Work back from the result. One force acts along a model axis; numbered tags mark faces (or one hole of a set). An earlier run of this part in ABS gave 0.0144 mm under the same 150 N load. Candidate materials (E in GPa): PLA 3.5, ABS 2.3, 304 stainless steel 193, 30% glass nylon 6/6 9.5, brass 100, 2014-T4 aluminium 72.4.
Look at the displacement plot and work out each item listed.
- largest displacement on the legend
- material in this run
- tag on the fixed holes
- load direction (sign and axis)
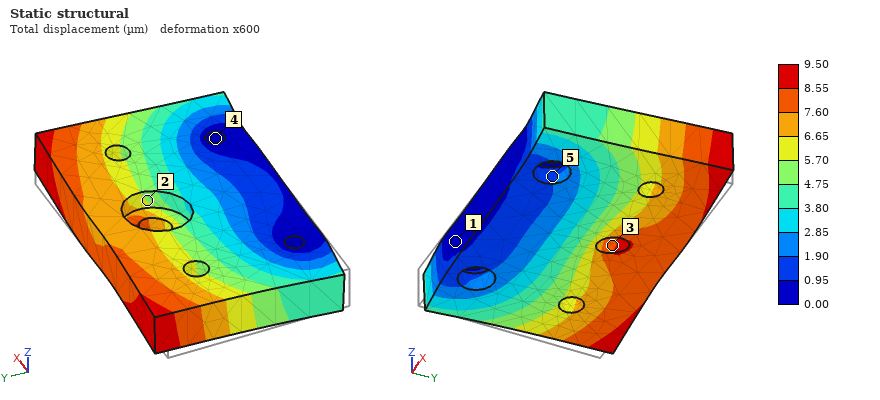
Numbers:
9.50 µm
PLA
4
+X
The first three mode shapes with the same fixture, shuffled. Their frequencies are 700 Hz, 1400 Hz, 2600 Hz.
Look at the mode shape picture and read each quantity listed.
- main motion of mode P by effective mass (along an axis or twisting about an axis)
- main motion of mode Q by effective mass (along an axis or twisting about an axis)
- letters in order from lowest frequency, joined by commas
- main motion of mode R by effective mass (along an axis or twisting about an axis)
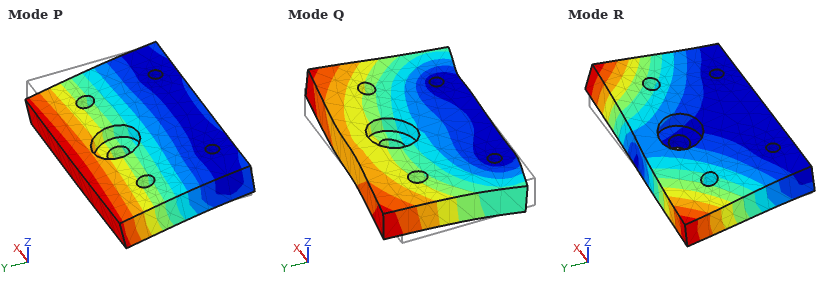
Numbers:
along Z
along X
P, R, Q
twisting about Y
